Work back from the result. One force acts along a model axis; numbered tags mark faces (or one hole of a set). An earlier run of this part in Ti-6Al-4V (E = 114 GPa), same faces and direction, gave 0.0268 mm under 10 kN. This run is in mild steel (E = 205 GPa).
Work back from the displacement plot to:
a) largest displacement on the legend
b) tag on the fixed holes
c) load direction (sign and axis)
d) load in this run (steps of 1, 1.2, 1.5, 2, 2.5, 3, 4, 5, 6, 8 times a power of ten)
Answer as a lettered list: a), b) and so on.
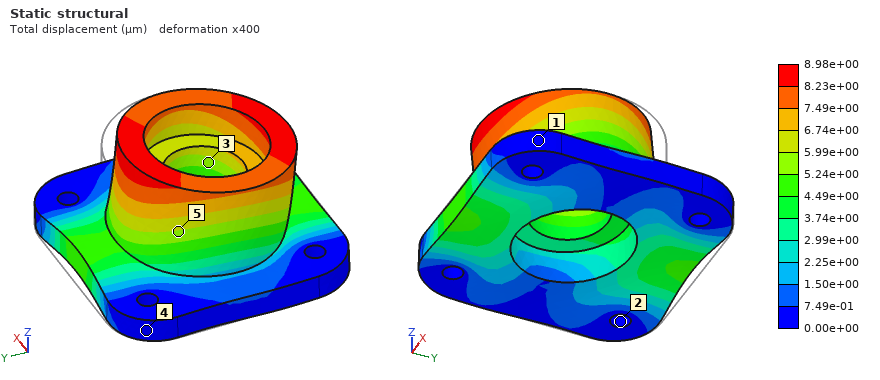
a) 8.98e+00 µm
b) 2
c) -Y
d) 6 kN
